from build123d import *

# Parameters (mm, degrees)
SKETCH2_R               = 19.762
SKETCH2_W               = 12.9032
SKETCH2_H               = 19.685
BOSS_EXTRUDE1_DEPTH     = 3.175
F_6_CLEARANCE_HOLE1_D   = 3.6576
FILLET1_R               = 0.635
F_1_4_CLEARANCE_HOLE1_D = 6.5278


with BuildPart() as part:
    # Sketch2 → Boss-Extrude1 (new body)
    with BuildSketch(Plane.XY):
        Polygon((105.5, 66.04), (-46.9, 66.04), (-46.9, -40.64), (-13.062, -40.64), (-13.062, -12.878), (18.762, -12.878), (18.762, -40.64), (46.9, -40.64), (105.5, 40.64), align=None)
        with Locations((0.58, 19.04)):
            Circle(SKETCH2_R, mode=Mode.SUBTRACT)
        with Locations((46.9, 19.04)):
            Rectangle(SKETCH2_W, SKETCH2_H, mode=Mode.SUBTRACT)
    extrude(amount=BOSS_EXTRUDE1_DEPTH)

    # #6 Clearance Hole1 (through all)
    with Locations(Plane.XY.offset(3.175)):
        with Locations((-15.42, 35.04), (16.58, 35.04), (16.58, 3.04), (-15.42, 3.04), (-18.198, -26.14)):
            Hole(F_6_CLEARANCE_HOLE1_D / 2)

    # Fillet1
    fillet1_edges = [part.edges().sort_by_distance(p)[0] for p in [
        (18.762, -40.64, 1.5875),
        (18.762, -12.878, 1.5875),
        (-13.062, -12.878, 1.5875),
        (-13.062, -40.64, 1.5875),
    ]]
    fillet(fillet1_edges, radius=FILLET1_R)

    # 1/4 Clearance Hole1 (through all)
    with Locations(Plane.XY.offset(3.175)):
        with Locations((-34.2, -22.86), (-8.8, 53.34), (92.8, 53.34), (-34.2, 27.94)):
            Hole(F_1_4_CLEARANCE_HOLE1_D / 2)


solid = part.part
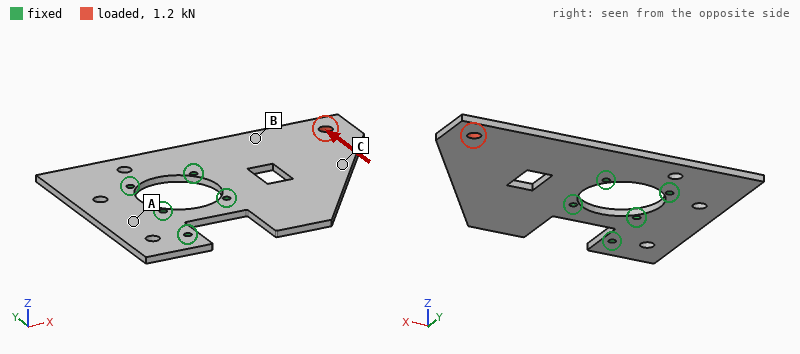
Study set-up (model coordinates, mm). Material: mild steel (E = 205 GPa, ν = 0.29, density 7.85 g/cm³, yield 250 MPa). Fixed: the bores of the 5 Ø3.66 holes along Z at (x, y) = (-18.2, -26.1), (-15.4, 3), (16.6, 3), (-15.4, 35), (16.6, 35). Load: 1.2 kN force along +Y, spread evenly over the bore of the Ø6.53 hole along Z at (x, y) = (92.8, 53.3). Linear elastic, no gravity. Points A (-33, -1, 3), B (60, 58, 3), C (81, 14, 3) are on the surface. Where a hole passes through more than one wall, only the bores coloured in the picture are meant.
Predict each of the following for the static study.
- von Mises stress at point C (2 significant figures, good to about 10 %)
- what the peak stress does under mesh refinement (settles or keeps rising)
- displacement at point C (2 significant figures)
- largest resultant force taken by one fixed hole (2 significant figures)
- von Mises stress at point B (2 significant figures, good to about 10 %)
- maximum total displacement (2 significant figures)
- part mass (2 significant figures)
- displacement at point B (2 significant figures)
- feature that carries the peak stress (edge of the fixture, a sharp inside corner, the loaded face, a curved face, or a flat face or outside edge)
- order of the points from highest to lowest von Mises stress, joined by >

18 MPa
keeps rising
18 µm
1.5 kN
9.7 MPa
30 µm
280 g
15 µm
edge of the fixture
C > B > A
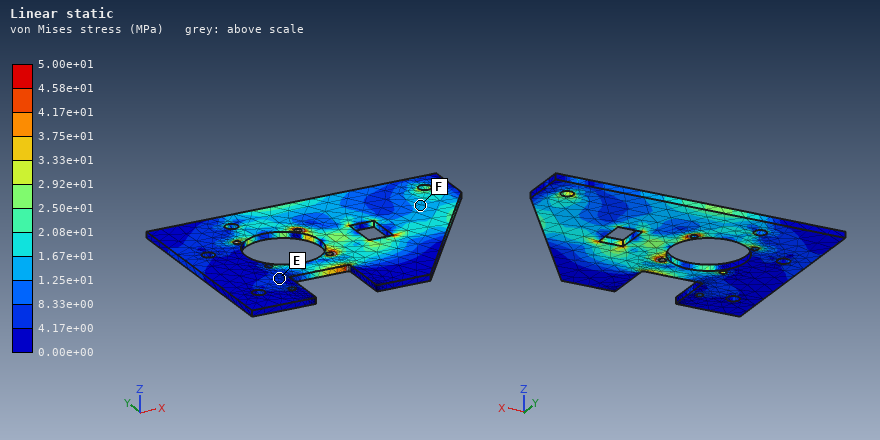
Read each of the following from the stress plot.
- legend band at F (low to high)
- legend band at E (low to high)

1.25e+01 to 1.67e+01 MPa
4.17e+00 to 8.33e+00 MPa
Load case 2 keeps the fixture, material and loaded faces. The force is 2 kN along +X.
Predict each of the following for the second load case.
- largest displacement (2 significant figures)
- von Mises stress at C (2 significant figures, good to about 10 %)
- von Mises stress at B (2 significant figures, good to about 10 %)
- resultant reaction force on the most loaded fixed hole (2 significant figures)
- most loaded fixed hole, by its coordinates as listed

20 µm
5.4 MPa
22 MPa
1.7 kN
(16.6, 35)
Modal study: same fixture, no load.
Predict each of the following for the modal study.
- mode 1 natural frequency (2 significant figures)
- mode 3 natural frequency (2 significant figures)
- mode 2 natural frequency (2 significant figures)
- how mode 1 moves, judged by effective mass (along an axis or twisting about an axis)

380 Hz
1500 Hz
890 Hz
along Z
